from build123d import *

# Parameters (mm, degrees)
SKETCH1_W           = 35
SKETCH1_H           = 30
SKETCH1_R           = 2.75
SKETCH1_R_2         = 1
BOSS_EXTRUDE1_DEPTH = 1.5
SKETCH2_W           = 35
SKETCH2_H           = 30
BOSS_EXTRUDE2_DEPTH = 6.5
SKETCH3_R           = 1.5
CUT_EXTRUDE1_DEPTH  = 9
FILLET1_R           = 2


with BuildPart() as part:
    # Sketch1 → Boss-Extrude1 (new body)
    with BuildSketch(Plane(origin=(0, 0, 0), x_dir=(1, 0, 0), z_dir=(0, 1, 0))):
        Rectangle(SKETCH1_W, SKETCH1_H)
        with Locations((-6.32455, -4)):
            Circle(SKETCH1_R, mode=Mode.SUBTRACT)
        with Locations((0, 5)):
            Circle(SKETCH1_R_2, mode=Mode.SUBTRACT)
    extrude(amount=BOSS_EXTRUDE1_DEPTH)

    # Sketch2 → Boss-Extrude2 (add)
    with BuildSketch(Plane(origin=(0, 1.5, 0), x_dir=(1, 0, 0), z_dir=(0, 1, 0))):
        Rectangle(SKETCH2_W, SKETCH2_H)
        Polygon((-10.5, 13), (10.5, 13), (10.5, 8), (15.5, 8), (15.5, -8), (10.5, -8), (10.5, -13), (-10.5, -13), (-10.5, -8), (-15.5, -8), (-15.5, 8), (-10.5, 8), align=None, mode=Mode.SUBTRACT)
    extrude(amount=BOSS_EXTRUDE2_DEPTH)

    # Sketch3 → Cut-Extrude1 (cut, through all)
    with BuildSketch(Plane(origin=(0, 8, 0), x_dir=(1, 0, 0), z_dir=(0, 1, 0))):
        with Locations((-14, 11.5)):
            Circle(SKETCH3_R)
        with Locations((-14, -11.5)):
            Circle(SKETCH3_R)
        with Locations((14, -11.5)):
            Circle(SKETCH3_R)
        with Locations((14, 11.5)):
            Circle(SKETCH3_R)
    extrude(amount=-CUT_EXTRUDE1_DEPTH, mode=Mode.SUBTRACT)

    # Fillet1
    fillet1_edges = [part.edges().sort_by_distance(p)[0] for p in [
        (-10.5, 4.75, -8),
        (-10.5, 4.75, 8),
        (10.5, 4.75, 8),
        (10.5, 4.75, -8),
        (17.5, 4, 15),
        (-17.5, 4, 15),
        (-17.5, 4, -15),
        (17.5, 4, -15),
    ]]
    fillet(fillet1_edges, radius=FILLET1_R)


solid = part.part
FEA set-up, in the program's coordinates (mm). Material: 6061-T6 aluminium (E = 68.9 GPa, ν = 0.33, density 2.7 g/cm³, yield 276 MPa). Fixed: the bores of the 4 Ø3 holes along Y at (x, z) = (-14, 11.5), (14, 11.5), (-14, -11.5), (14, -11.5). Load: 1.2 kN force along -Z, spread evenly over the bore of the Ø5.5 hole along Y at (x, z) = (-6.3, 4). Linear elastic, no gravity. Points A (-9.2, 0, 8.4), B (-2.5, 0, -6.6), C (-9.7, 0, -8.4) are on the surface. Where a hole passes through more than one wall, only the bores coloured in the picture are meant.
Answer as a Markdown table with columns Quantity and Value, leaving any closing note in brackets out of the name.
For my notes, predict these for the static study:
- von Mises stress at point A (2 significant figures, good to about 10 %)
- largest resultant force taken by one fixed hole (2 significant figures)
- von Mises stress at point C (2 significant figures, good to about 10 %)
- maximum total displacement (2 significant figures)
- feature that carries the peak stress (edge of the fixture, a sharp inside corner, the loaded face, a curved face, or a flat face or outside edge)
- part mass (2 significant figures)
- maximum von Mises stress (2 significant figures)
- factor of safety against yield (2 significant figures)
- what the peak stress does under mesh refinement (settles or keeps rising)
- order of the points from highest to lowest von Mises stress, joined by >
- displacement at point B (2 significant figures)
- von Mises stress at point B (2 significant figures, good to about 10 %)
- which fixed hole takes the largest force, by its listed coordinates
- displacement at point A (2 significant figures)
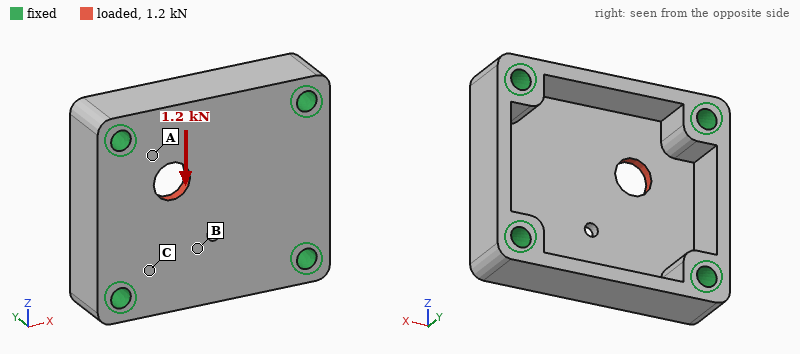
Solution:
| Quantity | Value |
|---|---|
| von Mises stress at point A | 42 MPa |
| largest resultant force taken by one fixed hole | 520 N |
| von Mises stress at point C | 24 MPa |
| maximum total displacement | 9.2 µm |
| feature that carries the peak stress | the loaded face |
| part mass | 9.4 g |
| maximum von Mises stress | 85 MPa |
| factor of safety against yield | 3.2 |
| what the peak stress does under mesh refinement | settles |
| order of the points from highest to lowest von Mises stress, joined by > | A > C > B |
| displacement at point B | 4.3 µm |
| von Mises stress at point B | 11 MPa |
| which fixed hole takes the largest force, by its listed coordinates | (-14, 11.5) |
| displacement at point A | 4.7 µm |
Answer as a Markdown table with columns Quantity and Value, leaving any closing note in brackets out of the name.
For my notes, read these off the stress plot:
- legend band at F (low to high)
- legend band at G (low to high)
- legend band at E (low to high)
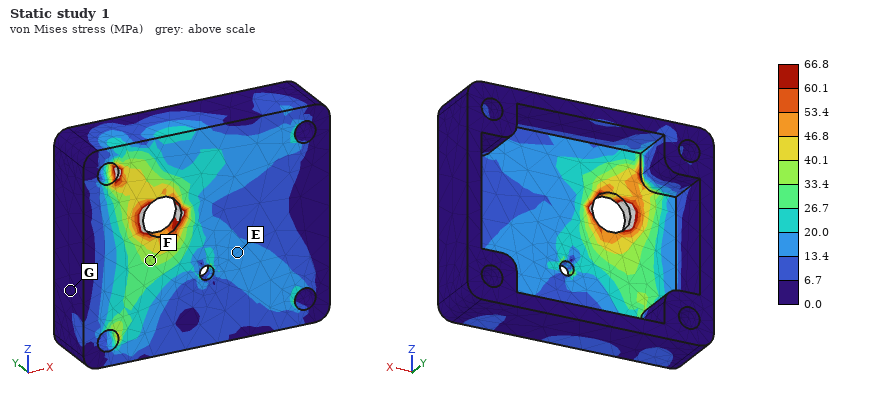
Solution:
| Quantity | Value |
|---|---|
| legend band at F | 33.4 to 40.1 MPa |
| legend band at G | 0.0 to 6.7 MPa |
| legend band at E | 13.4 to 20.0 MPa |
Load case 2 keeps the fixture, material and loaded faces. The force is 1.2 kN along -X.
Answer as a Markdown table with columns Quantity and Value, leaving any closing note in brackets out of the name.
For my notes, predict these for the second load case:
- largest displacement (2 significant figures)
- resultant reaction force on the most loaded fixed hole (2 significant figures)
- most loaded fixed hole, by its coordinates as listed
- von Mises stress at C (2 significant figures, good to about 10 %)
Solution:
| Quantity | Value |
|---|---|
| largest displacement | 8.4 µm |
| resultant reaction force on the most loaded fixed hole | 530 N |
| most loaded fixed hole, by its coordinates as listed | (-14, 11.5) |
| von Mises stress at C | 15 MPa |
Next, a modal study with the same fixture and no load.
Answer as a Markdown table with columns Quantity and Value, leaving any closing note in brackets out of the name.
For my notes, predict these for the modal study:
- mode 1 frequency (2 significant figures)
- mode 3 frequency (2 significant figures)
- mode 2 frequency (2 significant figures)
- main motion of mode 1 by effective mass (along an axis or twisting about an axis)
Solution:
| Quantity | Value |
|---|---|
| mode 1 frequency | 14 kHz |
| mode 3 frequency | 28 kHz |
| mode 2 frequency | 26 kHz |
| main motion of mode 1 by effective mass | along Y |
